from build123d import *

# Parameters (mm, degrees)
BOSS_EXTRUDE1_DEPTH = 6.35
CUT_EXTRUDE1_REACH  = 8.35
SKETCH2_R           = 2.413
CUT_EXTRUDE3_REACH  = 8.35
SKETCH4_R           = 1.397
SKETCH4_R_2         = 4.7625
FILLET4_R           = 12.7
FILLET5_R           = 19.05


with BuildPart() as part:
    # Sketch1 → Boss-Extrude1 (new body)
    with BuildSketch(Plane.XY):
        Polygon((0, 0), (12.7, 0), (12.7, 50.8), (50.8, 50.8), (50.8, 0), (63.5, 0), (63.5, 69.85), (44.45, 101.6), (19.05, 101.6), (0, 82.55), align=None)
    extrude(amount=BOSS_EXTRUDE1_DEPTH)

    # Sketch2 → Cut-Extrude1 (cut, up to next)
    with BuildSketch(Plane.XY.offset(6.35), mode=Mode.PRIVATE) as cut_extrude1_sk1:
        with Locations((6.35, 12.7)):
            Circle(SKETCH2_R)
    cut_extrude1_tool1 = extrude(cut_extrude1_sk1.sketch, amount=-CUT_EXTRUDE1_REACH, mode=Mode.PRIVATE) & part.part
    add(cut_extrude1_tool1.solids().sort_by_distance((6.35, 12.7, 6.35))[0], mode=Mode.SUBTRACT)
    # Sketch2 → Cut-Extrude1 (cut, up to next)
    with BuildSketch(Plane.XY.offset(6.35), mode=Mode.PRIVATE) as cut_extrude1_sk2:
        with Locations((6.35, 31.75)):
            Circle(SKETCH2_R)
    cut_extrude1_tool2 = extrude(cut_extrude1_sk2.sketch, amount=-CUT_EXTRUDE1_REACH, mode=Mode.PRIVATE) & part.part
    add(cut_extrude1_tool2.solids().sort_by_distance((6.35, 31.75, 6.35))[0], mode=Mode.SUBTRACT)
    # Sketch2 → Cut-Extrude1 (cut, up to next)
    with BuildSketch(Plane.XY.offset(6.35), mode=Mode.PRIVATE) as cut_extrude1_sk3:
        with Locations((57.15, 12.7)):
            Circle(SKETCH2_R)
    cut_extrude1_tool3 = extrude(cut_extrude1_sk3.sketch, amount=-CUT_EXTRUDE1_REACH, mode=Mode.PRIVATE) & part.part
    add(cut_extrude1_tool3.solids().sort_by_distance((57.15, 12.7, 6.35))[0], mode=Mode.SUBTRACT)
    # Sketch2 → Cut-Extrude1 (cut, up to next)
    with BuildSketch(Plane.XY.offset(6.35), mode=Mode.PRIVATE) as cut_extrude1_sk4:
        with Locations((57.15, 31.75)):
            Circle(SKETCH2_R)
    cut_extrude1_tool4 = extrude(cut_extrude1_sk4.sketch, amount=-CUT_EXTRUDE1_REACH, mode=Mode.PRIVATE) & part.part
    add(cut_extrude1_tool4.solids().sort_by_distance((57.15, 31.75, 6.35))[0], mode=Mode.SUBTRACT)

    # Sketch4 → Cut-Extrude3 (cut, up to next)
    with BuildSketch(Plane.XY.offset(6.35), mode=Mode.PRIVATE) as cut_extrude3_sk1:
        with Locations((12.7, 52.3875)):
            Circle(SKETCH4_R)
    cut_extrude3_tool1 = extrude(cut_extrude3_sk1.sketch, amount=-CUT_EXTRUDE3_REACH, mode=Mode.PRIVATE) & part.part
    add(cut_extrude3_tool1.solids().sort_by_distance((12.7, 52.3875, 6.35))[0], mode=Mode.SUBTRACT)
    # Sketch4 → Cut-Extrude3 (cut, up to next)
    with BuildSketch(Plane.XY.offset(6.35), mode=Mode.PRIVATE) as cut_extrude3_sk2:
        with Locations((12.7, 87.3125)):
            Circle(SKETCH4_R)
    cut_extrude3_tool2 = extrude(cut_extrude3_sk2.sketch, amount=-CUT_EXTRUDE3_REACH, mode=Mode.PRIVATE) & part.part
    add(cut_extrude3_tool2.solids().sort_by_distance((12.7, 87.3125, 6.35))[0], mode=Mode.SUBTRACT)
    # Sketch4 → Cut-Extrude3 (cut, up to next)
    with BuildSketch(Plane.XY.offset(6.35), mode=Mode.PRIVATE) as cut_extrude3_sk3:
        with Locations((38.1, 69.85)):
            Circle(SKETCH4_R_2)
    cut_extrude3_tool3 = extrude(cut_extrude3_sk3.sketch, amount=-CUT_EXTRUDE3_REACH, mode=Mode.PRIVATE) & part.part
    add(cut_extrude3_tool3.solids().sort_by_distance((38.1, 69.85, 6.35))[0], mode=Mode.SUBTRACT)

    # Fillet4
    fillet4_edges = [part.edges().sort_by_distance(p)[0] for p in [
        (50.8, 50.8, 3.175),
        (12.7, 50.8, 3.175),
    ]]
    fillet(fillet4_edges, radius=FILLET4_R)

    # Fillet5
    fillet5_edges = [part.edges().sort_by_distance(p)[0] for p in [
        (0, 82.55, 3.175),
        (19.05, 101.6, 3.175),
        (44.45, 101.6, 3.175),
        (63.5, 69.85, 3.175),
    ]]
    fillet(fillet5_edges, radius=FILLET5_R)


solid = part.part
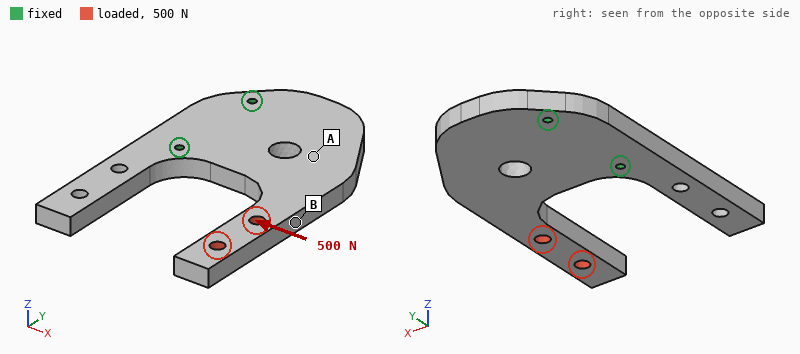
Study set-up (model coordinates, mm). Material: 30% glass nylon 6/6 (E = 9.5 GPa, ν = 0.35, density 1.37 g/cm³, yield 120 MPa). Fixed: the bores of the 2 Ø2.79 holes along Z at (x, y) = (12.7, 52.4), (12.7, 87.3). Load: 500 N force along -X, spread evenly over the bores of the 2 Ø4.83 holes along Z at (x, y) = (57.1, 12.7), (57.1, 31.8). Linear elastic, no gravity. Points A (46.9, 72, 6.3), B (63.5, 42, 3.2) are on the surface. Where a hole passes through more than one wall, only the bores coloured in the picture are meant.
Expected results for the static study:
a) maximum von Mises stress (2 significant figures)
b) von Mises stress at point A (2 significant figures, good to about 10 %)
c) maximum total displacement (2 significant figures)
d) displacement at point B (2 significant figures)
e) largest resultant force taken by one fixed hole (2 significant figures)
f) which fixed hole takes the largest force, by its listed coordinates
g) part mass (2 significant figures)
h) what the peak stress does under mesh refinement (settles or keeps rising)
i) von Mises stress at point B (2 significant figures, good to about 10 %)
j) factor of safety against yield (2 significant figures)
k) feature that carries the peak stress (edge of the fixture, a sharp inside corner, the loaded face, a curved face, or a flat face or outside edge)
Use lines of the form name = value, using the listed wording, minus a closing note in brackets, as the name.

maximum von Mises stress = 70 MPa
von Mises stress at point A = 8.6 MPa
maximum total displacement = 1.2 mm
displacement at point B = 0.26 mm
largest resultant force taken by one fixed hole = 930 N
which fixed hole takes the largest force, by its listed coordinates = (12.7, 52.4)
part mass = 34 g
what the peak stress does under mesh refinement = settles
von Mises stress at point B = 52 MPa
factor of safety against yield = 1.7
feature that carries the peak stress = a curved face
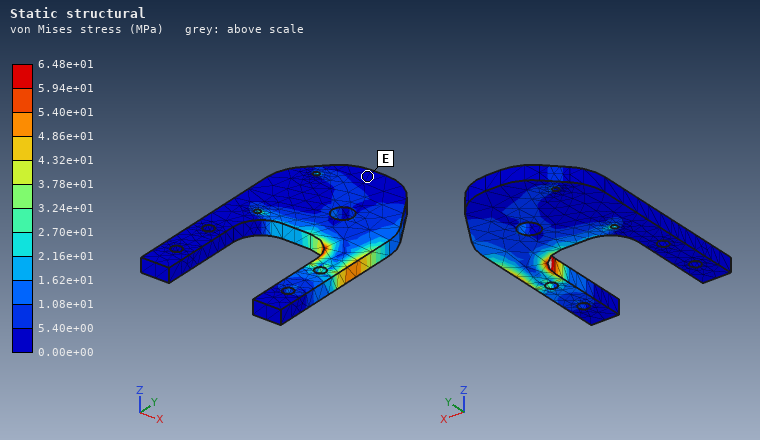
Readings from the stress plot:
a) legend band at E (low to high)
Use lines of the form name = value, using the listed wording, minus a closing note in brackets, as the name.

legend band at E = 0.00e+00 to 5.40e+00 MPa
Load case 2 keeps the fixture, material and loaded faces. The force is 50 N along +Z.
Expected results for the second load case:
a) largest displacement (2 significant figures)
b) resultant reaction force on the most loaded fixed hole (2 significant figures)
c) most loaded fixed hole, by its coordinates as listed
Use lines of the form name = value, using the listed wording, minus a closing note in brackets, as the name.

largest displacement = 1.3 mm
resultant reaction force on the most loaded fixed hole = 90 N
most loaded fixed hole, by its coordinates as listed = (12.7, 52.4)
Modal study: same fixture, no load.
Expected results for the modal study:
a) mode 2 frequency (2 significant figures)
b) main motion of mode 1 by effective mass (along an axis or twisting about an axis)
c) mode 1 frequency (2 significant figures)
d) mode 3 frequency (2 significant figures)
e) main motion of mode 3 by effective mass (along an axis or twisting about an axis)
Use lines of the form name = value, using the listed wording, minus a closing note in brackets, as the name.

mode 2 frequency = 970 Hz
main motion of mode 1 by effective mass = along Z
mode 1 frequency = 510 Hz
mode 3 frequency = 1100 Hz
main motion of mode 3 by effective mass = along Z
